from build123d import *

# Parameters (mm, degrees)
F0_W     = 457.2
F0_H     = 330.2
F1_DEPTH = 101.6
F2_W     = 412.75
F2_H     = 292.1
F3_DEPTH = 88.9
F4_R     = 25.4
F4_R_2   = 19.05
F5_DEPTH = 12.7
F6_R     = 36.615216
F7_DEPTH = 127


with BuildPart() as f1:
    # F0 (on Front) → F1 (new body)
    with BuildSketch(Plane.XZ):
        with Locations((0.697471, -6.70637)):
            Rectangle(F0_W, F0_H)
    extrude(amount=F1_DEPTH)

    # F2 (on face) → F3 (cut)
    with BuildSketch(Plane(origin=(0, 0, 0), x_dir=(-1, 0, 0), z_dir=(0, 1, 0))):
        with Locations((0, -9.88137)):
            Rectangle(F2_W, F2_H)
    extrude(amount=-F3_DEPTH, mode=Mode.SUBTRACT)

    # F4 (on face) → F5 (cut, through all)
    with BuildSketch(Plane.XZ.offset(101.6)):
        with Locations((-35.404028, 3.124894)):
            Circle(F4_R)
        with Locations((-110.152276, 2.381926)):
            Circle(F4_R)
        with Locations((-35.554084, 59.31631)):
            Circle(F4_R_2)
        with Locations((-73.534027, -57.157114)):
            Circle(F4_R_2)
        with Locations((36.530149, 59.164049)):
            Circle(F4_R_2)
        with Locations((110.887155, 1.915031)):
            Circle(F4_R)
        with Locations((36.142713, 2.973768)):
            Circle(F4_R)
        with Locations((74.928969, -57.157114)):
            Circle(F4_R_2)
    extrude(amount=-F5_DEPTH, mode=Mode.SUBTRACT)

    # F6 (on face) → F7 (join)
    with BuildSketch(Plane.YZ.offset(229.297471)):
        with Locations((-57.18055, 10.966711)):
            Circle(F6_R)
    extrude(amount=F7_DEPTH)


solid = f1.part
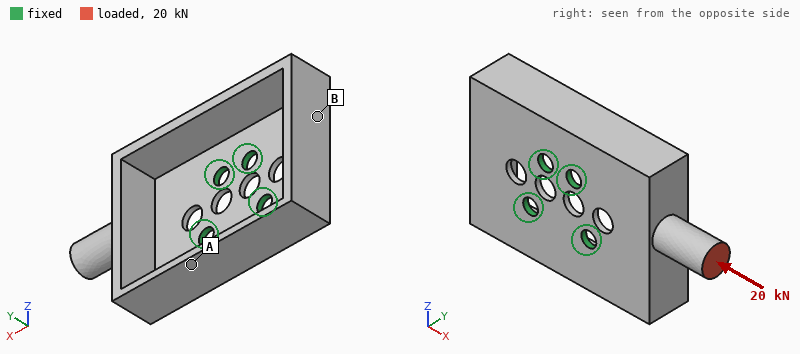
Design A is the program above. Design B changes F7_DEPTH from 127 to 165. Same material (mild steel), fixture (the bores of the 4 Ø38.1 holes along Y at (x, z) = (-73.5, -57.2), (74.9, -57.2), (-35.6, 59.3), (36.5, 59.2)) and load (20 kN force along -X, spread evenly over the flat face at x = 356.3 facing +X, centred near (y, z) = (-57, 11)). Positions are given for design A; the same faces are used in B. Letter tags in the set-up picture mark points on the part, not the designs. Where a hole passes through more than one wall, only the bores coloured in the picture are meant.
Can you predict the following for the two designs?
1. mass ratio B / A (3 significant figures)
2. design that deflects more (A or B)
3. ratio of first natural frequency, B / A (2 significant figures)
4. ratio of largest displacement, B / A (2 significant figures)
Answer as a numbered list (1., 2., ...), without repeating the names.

1. 1.03
2. B
3. 0.91
4. 1.2
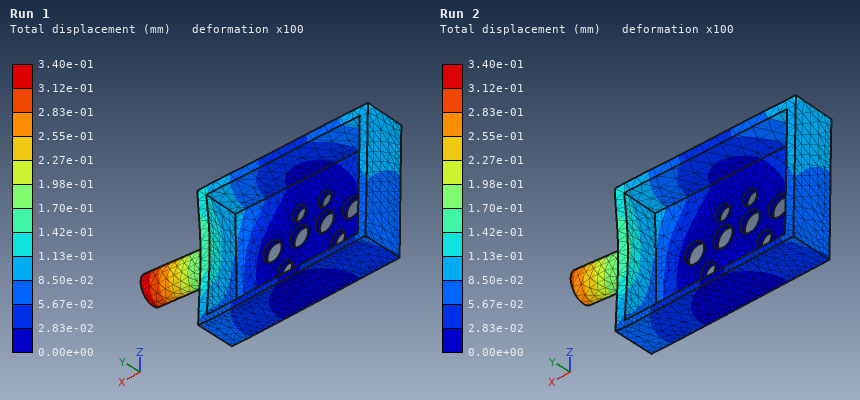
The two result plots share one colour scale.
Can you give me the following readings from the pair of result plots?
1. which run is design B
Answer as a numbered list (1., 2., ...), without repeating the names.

1. Run 1
